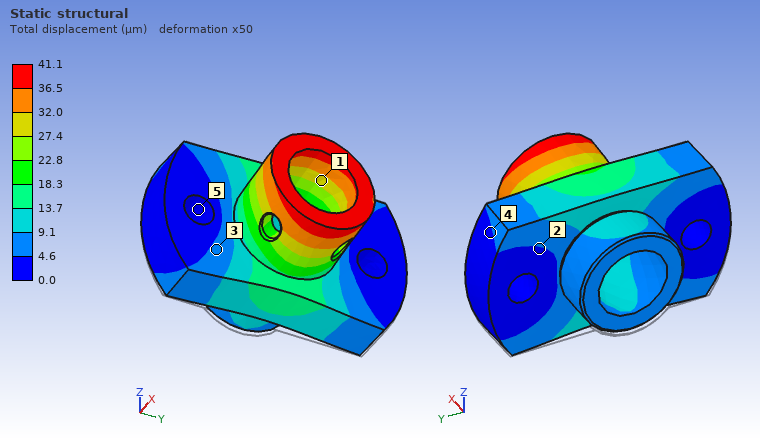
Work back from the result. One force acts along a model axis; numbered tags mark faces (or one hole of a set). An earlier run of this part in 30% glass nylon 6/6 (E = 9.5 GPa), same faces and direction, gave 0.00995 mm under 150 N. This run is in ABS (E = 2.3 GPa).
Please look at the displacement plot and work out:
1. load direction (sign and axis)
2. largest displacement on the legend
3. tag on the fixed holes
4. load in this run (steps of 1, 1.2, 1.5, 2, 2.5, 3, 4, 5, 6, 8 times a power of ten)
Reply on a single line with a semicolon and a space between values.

+Z; 41.1 µm; 5; 150 N
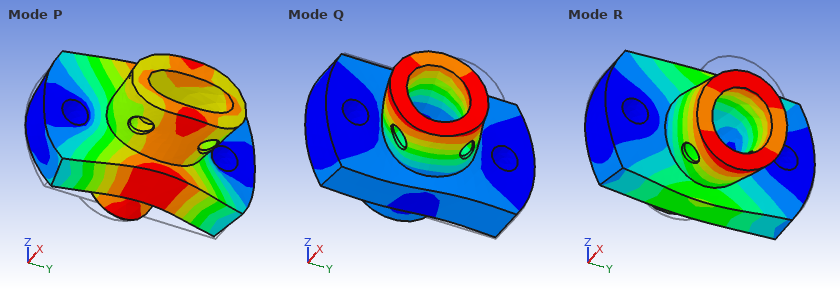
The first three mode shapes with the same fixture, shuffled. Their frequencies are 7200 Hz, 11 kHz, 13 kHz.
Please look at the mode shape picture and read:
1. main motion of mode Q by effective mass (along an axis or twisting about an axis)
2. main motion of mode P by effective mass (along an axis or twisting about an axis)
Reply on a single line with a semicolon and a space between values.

along Y; along X
